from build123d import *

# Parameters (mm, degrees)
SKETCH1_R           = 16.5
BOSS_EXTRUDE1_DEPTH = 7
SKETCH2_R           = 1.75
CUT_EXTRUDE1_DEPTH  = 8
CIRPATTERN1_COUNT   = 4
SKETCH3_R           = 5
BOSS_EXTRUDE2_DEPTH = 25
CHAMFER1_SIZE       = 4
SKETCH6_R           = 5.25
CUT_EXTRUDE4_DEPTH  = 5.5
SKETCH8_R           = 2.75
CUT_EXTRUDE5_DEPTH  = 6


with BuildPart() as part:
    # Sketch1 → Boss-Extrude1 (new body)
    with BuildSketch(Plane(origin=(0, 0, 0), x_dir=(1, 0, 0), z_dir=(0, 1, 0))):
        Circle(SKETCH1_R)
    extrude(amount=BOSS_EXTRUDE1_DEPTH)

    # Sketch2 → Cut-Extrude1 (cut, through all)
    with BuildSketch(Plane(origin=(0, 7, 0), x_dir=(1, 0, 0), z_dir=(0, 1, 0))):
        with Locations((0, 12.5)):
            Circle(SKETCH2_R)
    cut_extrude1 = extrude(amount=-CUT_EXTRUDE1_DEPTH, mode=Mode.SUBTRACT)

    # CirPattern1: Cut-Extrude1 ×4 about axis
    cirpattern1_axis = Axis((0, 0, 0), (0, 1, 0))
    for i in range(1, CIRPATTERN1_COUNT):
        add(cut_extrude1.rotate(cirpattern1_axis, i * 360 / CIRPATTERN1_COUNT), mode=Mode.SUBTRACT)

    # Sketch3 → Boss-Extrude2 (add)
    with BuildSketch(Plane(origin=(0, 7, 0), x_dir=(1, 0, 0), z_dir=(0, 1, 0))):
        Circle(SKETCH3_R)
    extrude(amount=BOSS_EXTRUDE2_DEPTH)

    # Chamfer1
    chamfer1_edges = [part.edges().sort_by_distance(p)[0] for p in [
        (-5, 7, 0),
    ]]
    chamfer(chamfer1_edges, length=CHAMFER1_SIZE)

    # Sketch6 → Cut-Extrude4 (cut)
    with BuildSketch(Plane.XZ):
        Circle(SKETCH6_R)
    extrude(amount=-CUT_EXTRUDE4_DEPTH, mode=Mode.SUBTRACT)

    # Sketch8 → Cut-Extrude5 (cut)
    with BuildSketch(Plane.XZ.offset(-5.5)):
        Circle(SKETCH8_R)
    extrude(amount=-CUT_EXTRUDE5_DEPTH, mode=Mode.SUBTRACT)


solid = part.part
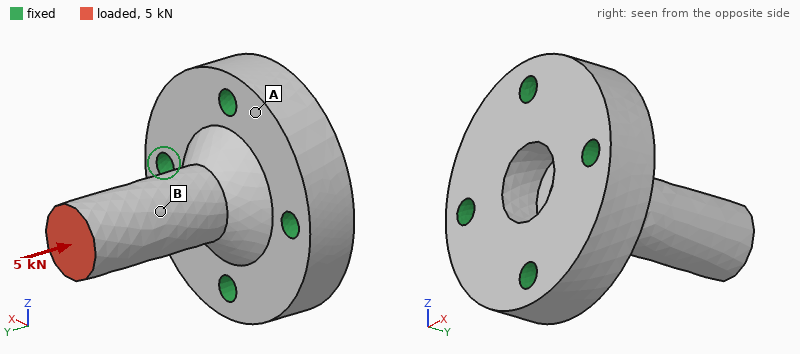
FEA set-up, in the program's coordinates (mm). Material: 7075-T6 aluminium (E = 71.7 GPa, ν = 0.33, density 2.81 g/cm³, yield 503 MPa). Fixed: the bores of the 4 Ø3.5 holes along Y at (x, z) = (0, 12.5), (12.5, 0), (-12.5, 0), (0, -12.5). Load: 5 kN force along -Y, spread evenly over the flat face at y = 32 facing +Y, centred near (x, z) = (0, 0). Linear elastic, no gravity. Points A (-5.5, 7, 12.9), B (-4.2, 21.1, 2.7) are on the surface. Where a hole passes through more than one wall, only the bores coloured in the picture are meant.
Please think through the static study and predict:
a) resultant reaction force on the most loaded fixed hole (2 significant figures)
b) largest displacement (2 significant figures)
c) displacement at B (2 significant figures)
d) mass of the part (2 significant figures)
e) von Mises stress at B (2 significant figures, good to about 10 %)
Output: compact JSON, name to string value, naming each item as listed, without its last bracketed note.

{"resultant reaction force on the most loaded fixed hole": "1.4 kN", "largest displacement": "28 µm", "displacement at B": "19 µm", "mass of the part": "21 g", "von Mises stress at B": "63 MPa"}
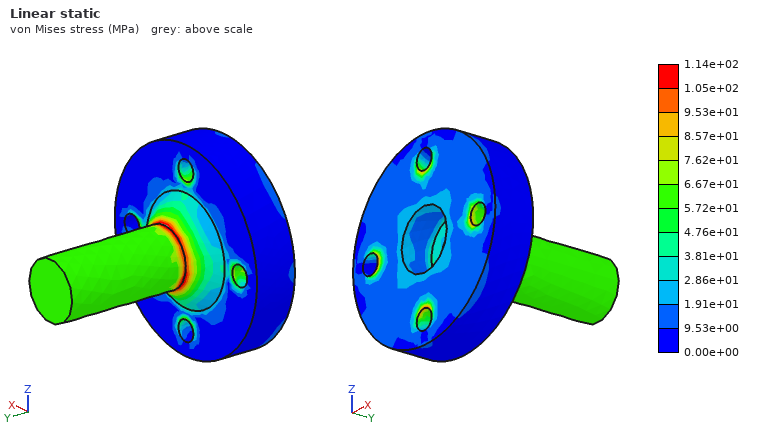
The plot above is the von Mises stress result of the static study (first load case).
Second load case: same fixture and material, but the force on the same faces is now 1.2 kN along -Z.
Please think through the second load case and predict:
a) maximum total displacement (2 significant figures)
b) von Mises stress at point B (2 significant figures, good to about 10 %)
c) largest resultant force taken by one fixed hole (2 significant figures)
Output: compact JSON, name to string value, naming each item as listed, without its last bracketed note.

{"maximum total displacement": "0.19 mm", "von Mises stress at point B": "78 MPa", "largest resultant force taken by one fixed hole": "1.6 kN"}
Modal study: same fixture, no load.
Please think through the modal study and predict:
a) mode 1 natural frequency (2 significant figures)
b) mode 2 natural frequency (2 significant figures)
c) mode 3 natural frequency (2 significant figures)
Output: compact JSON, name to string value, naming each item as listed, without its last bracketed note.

{"mode 1 natural frequency": "11 kHz", "mode 2 natural frequency": "11 kHz", "mode 3 natural frequency": "33 kHz"}
